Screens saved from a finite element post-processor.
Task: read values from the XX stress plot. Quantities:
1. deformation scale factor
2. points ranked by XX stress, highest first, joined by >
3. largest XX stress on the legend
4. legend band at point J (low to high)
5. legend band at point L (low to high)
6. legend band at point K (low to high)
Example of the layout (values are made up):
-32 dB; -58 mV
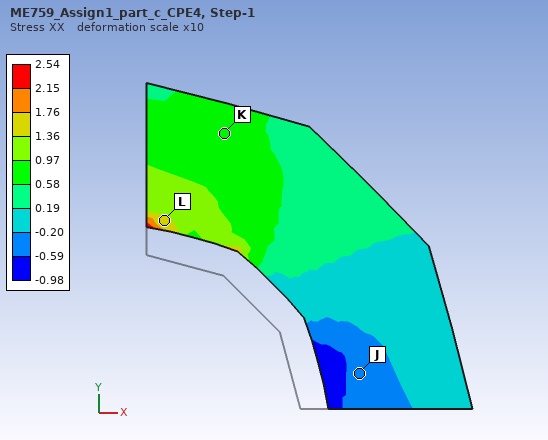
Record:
10; L > K > J; 2.54; -0.59 to -0.20; 1.36 to 1.76; 0.58 to 0.97
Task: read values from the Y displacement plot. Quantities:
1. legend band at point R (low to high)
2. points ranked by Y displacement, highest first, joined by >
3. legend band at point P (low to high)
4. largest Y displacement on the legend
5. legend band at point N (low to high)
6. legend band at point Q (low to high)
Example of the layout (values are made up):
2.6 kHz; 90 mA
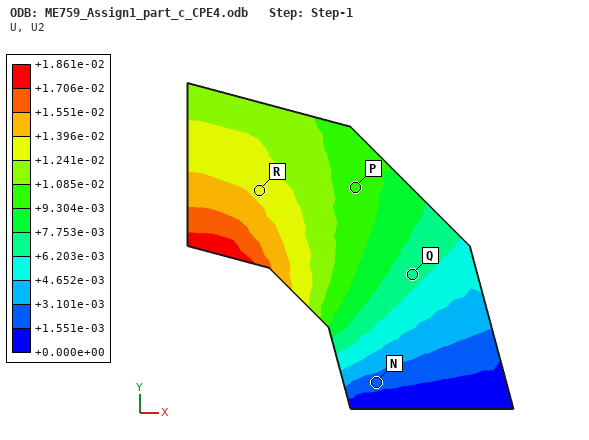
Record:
+1.241e-02 to +1.396e-02; R > P > Q > N; +9.304e-03 to +1.085e-02; +1.861e-02; +1.551e-03 to +3.101e-03; +6.203e-03 to +7.753e-03
